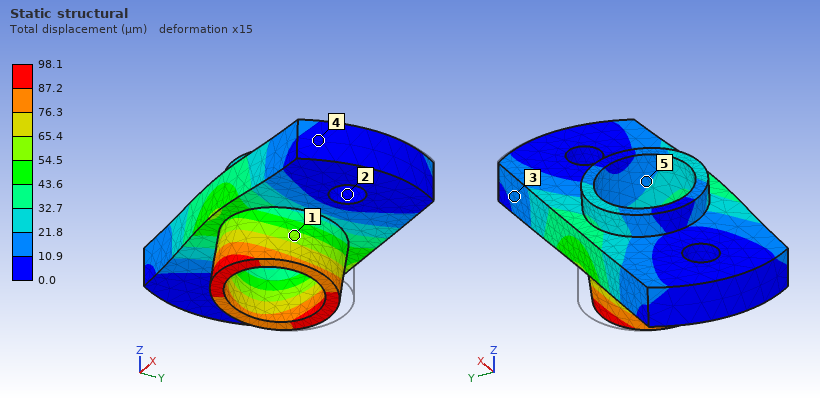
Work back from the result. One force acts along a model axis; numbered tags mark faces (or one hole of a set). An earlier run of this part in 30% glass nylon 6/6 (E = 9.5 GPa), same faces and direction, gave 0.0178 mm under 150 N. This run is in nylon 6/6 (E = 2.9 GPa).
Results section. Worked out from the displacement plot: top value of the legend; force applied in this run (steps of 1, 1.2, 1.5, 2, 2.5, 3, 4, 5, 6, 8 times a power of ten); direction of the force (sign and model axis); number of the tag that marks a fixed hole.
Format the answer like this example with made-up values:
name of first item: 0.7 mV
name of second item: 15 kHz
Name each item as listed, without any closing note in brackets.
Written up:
top value of the legend: 98.1 µm
force applied in this run: 250 N
direction of the force: -Y
number of the tag that marks a fixed hole: 2
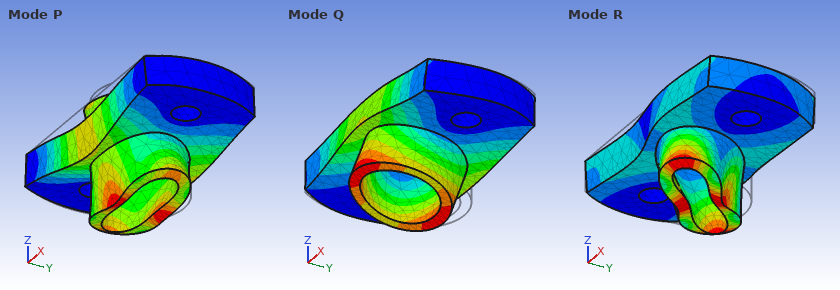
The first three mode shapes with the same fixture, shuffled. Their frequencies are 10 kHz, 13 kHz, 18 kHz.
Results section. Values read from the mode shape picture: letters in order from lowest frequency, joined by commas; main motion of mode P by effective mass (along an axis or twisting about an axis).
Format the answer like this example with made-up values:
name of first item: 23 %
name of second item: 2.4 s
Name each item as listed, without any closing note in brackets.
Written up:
letters in order from lowest frequency, joined by commas: Q, P, R
main motion of mode P by effective mass: along Z
